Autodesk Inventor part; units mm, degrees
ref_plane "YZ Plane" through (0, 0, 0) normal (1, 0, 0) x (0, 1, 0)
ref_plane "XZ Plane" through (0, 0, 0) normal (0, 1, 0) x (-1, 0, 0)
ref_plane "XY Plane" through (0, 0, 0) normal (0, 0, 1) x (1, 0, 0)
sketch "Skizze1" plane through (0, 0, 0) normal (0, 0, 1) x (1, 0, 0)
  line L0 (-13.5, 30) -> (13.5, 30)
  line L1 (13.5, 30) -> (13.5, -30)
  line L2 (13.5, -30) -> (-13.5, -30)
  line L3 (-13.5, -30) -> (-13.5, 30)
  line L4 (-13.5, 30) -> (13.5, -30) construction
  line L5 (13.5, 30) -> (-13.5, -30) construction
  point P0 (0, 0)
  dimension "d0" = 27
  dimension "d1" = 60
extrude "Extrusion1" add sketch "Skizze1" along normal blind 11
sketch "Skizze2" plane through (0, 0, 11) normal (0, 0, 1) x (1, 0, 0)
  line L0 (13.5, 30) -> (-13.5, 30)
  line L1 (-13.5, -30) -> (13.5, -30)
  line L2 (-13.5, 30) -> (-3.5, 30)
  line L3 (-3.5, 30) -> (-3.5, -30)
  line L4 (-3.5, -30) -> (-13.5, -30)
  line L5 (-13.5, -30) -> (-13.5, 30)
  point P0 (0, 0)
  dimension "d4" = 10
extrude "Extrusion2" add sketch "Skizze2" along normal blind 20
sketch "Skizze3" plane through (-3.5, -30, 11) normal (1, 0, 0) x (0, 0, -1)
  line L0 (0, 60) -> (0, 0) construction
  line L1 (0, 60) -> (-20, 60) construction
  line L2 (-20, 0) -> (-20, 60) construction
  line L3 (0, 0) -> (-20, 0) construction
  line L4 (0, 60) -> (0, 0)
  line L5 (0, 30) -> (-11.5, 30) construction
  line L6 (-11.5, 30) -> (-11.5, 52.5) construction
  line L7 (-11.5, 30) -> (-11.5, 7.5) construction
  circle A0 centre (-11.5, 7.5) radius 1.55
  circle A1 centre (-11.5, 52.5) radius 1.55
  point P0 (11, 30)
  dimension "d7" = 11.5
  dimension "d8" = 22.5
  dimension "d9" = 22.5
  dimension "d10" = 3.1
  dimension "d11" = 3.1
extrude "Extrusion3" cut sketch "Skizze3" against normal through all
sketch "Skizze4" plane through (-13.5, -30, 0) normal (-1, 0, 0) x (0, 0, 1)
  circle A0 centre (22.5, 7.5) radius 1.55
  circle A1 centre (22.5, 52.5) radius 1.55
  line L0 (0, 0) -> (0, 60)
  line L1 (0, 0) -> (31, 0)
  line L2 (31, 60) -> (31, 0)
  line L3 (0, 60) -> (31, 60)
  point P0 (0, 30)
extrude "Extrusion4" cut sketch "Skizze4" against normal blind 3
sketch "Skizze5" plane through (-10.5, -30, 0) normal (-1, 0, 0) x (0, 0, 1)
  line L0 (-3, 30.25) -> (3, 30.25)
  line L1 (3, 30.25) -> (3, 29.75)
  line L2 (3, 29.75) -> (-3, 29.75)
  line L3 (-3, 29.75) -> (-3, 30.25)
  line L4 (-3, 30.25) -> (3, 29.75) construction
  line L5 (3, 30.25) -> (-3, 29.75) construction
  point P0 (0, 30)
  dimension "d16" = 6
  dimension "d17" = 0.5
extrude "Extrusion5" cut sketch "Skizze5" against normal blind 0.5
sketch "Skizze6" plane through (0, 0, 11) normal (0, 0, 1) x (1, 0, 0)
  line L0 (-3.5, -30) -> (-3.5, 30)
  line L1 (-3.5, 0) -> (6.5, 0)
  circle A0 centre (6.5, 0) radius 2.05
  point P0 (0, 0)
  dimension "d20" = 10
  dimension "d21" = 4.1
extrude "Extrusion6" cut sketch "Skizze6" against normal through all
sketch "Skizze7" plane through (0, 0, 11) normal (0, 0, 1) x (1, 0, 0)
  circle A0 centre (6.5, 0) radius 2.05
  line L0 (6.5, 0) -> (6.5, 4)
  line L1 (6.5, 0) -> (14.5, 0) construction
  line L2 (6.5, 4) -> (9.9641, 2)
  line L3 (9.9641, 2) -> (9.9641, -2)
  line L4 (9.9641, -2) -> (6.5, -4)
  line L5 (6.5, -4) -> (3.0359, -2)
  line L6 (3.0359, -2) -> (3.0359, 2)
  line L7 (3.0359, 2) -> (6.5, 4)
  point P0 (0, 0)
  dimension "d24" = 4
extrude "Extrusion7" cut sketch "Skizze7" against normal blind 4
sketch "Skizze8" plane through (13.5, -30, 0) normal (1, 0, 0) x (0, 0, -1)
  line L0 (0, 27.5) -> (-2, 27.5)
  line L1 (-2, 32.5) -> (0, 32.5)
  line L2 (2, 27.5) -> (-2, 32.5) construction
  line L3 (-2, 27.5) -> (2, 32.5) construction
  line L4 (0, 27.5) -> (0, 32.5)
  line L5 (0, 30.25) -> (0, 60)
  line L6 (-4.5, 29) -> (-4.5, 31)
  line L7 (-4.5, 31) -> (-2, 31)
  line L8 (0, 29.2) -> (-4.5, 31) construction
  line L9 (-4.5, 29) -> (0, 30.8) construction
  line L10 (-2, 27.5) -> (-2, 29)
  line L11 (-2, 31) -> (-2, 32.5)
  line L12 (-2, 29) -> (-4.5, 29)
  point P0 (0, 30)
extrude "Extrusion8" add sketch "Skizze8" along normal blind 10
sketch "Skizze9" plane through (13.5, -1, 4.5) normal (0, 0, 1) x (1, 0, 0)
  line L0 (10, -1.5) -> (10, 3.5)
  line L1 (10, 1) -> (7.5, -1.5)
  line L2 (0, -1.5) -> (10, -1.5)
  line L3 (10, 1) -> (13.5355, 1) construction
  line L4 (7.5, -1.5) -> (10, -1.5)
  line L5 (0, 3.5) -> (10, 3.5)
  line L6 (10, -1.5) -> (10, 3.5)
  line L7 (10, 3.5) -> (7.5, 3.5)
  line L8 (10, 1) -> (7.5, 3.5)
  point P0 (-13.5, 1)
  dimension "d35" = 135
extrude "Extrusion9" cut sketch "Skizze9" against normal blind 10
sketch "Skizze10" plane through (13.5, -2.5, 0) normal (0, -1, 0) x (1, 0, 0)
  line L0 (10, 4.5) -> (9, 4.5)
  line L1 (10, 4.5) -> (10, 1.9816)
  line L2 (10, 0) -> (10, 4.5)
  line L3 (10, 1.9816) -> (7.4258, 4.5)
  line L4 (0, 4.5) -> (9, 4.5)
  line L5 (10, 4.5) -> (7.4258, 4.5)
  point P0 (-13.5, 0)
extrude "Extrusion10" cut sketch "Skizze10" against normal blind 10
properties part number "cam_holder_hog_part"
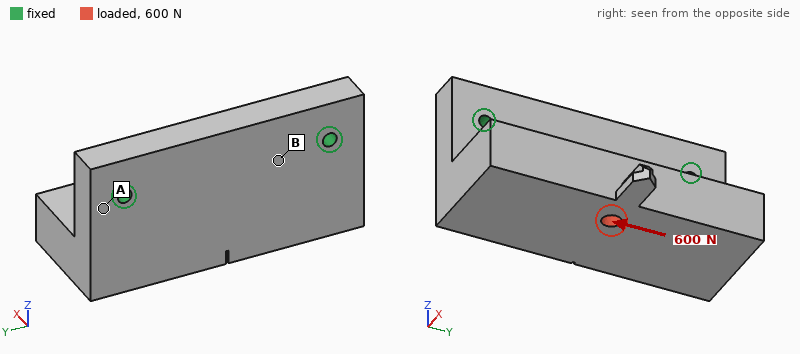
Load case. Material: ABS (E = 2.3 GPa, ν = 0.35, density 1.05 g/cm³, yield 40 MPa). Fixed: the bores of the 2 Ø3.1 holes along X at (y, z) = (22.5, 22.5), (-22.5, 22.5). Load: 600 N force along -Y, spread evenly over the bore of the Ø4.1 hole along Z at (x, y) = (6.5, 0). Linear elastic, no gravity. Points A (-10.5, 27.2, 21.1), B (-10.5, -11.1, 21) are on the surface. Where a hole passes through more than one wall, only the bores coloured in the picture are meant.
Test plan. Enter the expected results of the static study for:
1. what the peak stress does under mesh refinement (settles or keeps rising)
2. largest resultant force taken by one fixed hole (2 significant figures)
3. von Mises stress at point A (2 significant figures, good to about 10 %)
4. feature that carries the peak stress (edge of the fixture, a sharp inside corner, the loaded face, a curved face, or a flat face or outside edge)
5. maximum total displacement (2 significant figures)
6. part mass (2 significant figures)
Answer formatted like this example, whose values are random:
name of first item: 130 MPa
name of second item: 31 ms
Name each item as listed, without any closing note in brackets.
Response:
what the peak stress does under mesh refinement: keeps rising
largest resultant force taken by one fixed hole: 420 N
von Mises stress at point A: 6.2 MPa
feature that carries the peak stress: edge of the fixture
maximum total displacement: 0.20 mm
part mass: 25 g
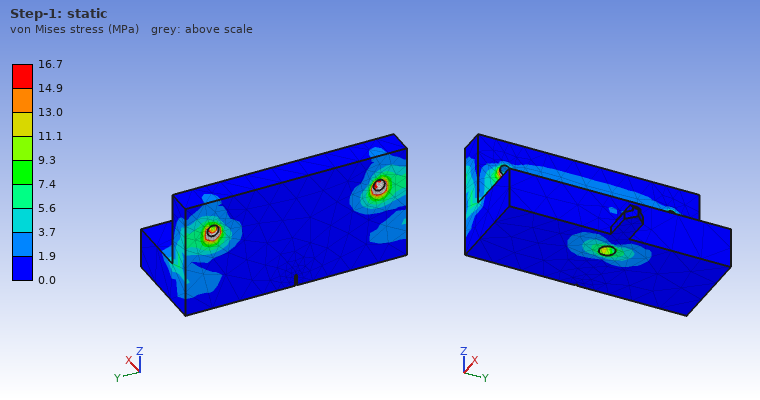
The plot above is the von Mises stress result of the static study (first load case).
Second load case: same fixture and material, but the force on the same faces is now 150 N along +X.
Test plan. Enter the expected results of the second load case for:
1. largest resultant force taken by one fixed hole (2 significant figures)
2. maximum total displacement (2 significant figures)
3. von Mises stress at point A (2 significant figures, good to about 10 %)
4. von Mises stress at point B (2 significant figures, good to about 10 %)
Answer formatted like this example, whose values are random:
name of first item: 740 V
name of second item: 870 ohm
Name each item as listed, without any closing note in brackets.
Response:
largest resultant force taken by one fixed hole: 75 N
maximum total displacement: 0.40 mm
von Mises stress at point A: 4.7 MPa
von Mises stress at point B: 2.4 MPa
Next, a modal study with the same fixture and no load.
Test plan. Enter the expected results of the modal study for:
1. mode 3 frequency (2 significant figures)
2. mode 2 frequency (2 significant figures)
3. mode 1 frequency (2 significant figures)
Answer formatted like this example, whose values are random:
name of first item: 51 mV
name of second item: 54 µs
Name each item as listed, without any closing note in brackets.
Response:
mode 3 frequency: 3400 Hz
mode 2 frequency: 2200 Hz
mode 1 frequency: 1000 Hz
